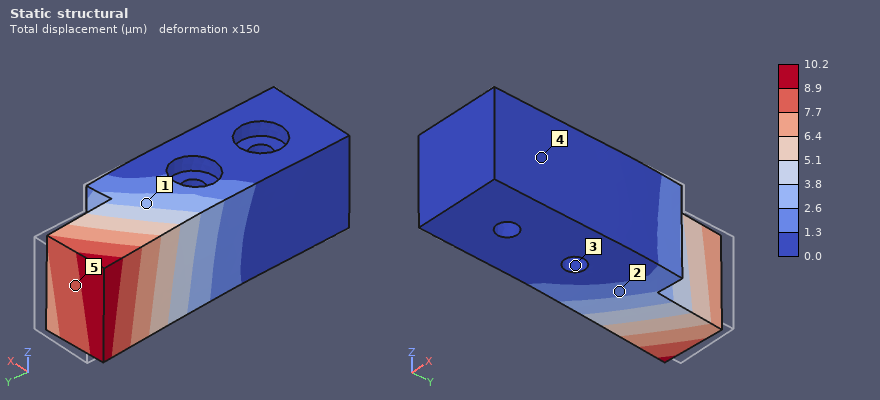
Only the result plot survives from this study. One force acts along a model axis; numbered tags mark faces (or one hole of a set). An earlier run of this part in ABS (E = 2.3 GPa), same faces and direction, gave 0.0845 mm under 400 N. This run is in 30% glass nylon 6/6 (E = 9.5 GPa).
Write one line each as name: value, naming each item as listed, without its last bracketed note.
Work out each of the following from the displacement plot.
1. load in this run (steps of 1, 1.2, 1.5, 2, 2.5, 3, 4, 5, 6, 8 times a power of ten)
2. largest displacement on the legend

load in this run: 200 N
largest displacement on the legend: 10.2 µm
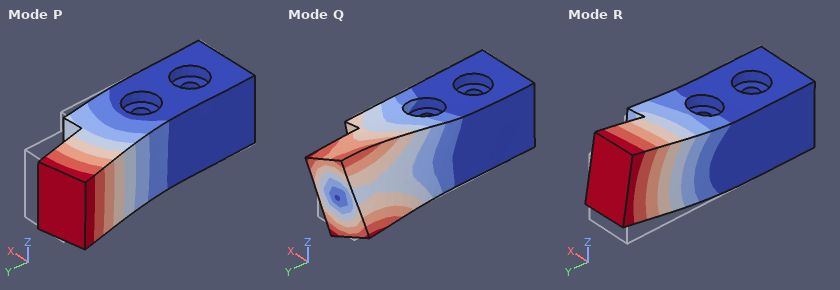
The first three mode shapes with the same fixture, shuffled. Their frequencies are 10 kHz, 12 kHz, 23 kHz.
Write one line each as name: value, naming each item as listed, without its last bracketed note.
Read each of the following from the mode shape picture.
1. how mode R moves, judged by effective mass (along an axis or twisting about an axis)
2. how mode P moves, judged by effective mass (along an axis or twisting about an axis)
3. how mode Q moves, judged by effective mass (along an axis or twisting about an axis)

how mode R moves, judged by effective mass: along Z
how mode P moves, judged by effective mass: along X
how mode Q moves, judged by effective mass: twisting about Y
